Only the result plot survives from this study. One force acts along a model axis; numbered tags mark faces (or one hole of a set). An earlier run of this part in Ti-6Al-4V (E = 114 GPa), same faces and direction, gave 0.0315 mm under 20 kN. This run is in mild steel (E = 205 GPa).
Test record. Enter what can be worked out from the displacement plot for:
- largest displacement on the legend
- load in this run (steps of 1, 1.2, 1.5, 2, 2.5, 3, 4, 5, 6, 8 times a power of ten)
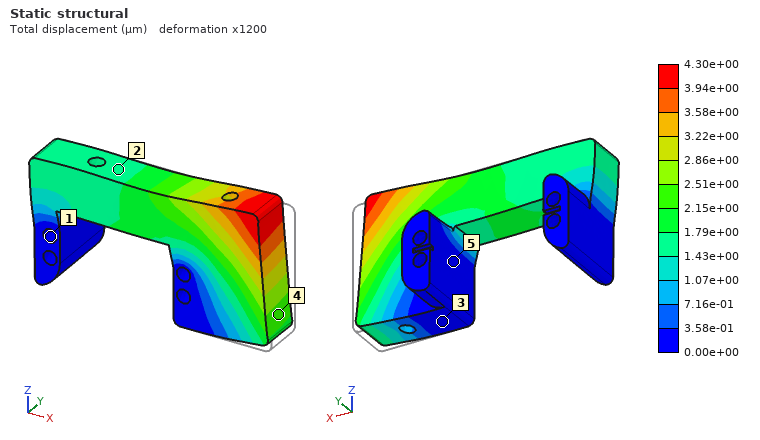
4.30e+00 µm
5 kN
